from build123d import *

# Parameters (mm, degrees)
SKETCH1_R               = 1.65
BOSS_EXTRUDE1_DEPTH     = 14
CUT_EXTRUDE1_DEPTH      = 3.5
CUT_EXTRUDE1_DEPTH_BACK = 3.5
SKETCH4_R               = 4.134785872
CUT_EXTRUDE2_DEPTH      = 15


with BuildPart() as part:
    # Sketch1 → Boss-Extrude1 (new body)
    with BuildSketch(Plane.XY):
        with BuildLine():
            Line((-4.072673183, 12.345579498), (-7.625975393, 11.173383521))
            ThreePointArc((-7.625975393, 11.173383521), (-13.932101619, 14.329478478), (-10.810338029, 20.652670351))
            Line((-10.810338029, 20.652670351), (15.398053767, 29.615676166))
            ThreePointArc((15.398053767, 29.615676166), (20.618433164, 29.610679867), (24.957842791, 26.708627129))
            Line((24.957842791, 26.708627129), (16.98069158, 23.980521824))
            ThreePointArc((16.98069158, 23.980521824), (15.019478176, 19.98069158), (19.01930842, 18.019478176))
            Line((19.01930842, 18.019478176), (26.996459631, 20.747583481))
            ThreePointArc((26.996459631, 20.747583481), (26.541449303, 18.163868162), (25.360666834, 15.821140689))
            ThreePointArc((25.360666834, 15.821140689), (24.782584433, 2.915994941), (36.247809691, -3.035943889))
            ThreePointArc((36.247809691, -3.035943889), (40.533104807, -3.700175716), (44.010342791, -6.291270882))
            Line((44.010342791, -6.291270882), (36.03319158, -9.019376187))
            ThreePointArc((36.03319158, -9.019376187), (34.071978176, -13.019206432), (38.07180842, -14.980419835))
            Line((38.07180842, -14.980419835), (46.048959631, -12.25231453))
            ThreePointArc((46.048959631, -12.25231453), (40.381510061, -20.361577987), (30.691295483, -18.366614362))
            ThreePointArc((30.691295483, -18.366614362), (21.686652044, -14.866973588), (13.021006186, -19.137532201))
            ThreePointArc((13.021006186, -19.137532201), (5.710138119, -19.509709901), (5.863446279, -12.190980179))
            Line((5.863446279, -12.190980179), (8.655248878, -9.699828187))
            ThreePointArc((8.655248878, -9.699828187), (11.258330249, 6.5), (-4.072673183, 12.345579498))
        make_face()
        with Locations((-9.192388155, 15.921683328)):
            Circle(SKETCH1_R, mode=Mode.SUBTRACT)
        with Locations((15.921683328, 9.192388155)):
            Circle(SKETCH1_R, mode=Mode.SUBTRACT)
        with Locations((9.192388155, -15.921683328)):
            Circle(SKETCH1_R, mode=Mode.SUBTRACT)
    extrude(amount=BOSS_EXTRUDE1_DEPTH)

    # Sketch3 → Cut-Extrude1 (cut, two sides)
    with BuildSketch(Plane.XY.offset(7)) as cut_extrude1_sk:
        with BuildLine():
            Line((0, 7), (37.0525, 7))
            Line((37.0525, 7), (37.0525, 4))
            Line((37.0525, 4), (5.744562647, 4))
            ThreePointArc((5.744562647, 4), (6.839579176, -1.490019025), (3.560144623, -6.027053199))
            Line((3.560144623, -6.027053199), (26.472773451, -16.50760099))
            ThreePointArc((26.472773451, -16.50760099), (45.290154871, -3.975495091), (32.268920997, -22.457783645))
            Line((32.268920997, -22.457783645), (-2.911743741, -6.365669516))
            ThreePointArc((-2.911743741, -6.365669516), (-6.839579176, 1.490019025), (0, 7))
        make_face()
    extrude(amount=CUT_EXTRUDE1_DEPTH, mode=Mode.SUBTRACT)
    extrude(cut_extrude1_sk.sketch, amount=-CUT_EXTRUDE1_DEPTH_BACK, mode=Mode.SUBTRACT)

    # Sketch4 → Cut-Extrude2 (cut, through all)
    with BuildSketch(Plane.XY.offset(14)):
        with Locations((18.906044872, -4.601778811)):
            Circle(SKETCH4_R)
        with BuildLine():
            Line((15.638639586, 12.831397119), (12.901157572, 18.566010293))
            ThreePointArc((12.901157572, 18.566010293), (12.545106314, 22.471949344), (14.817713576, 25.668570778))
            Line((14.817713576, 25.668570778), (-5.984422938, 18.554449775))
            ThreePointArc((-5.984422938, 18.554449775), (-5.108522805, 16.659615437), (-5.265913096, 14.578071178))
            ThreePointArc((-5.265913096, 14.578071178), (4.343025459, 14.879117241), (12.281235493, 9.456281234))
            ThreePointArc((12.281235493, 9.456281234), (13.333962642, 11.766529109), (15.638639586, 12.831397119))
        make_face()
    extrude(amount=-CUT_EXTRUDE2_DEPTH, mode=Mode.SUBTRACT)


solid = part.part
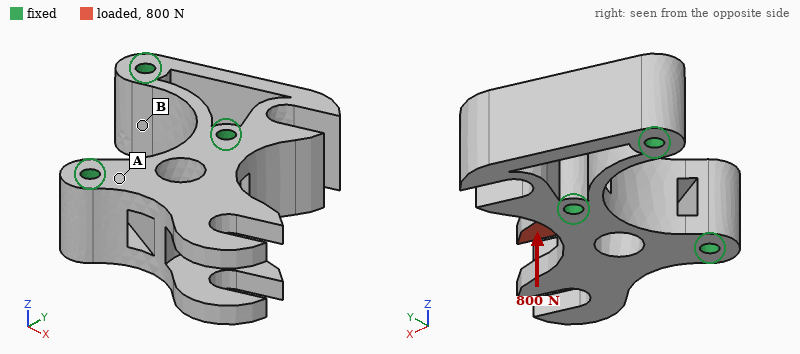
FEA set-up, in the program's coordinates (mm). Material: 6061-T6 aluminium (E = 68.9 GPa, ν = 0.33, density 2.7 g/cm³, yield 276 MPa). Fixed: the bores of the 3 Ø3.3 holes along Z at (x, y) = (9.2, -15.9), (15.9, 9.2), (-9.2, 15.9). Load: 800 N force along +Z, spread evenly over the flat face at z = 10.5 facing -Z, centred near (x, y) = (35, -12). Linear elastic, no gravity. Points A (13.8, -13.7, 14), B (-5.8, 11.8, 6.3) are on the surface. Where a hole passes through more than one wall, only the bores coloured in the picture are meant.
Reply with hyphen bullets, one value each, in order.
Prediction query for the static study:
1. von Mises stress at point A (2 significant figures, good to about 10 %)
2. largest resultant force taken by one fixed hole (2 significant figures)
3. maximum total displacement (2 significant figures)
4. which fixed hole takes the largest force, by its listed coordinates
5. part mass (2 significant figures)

- 54 MPa
- 450 N
- 0.37 mm
- (9.2, -15.9)
- 30 g
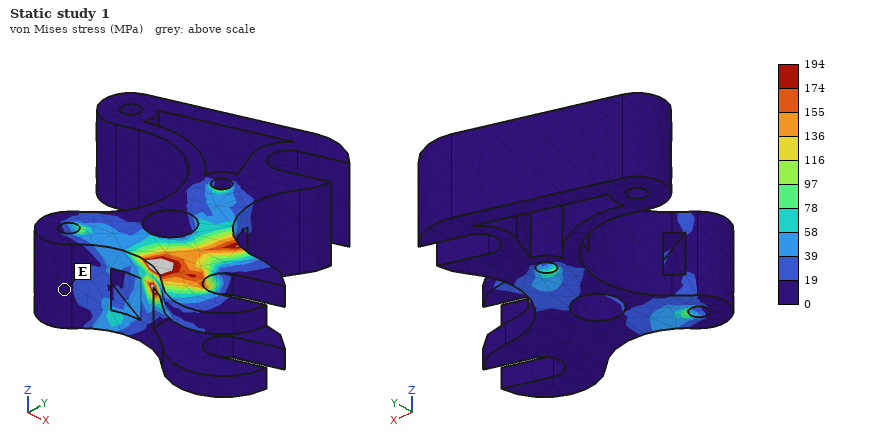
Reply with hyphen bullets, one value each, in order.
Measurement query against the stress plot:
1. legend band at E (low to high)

- 0 to 19 MPa
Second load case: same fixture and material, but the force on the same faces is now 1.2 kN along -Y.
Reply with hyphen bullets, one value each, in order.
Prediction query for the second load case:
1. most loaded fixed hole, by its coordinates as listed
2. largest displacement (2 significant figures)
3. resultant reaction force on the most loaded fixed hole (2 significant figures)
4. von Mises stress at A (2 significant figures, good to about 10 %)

- (15.9, 9.2)
- 0.14 mm
- 1.4 kN
- 25 MPa
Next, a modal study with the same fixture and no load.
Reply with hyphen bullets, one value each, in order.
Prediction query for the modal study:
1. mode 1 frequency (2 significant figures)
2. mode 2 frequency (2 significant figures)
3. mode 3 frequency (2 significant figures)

- 6400 Hz
- 7000 Hz
- 13 kHz
